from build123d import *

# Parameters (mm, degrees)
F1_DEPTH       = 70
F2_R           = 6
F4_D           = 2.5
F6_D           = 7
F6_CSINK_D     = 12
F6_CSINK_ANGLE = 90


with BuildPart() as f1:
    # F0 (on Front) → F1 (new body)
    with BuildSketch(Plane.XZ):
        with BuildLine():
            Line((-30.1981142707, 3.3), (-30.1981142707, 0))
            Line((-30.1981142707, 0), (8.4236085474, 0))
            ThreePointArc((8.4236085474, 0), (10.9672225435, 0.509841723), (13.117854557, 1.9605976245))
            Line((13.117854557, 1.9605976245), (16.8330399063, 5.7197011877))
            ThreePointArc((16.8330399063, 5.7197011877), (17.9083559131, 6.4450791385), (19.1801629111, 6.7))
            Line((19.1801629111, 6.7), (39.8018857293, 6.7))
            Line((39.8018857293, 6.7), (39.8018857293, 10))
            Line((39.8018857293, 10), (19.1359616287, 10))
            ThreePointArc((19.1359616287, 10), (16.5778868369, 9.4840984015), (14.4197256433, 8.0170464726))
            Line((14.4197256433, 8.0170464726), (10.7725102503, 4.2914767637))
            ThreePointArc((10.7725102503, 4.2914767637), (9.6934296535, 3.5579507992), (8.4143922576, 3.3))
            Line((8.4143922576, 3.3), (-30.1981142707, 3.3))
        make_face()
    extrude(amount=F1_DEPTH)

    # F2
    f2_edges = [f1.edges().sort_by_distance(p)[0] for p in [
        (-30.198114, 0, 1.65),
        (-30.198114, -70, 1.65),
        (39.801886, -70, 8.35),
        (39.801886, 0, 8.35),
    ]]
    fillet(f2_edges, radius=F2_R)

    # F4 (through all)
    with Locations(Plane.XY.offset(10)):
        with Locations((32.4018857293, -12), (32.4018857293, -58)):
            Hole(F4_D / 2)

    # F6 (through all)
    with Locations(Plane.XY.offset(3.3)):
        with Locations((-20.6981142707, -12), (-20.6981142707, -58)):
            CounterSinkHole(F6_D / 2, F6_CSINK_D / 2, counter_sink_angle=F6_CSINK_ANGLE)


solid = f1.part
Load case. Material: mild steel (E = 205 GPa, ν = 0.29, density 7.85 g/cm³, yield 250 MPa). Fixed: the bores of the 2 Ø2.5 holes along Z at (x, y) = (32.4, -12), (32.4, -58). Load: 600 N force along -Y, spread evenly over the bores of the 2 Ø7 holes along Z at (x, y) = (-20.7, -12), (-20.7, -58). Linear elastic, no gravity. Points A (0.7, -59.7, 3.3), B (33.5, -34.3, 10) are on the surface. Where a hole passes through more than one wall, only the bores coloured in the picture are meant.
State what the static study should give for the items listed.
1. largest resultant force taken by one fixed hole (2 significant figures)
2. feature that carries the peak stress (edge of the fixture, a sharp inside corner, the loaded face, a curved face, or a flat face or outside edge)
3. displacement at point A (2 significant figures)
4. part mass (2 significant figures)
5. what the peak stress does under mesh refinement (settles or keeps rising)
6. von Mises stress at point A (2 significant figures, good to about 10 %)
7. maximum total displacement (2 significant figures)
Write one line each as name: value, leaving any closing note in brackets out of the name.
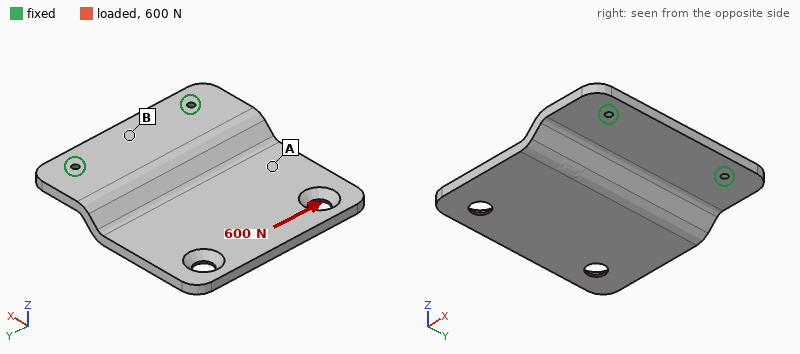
largest resultant force taken by one fixed hole: 750 N
feature that carries the peak stress: edge of the fixture
displacement at point A: 12 µm
part mass: 130 g
what the peak stress does under mesh refinement: keeps rising
von Mises stress at point A: 14 MPa
maximum total displacement: 22 µm
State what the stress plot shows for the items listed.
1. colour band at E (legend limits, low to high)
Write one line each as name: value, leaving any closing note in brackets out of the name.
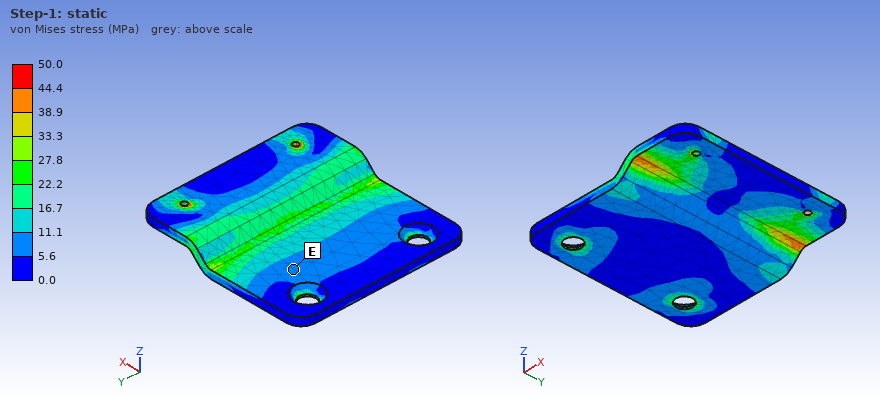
colour band at E: 5.6 to 11.1 MPa
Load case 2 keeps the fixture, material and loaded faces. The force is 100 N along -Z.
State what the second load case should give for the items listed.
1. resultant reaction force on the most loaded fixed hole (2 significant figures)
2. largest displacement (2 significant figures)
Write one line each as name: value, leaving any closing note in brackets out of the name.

resultant reaction force on the most loaded fixed hole: 52 N
largest displacement: 0.19 mm
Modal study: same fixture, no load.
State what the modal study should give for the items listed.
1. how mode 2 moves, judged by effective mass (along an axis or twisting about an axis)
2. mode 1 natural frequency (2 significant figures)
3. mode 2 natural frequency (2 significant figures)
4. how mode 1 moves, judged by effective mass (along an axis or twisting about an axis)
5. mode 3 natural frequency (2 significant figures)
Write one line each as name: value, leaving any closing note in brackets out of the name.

how mode 2 moves, judged by effective mass: twisting about X
mode 1 natural frequency: 620 Hz
mode 2 natural frequency: 1600 Hz
how mode 1 moves, judged by effective mass: along Z
mode 3 natural frequency: 3600 Hz
